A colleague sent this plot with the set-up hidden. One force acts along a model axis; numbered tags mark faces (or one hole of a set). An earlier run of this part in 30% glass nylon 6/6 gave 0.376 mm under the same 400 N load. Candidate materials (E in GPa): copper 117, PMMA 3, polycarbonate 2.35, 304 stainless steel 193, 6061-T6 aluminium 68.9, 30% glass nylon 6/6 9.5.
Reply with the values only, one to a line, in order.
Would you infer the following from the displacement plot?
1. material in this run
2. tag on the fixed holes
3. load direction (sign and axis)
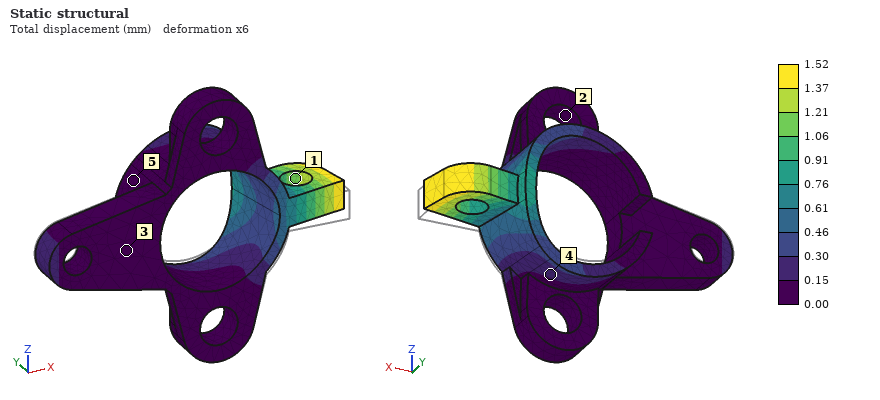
polycarbonate
2
+Y
